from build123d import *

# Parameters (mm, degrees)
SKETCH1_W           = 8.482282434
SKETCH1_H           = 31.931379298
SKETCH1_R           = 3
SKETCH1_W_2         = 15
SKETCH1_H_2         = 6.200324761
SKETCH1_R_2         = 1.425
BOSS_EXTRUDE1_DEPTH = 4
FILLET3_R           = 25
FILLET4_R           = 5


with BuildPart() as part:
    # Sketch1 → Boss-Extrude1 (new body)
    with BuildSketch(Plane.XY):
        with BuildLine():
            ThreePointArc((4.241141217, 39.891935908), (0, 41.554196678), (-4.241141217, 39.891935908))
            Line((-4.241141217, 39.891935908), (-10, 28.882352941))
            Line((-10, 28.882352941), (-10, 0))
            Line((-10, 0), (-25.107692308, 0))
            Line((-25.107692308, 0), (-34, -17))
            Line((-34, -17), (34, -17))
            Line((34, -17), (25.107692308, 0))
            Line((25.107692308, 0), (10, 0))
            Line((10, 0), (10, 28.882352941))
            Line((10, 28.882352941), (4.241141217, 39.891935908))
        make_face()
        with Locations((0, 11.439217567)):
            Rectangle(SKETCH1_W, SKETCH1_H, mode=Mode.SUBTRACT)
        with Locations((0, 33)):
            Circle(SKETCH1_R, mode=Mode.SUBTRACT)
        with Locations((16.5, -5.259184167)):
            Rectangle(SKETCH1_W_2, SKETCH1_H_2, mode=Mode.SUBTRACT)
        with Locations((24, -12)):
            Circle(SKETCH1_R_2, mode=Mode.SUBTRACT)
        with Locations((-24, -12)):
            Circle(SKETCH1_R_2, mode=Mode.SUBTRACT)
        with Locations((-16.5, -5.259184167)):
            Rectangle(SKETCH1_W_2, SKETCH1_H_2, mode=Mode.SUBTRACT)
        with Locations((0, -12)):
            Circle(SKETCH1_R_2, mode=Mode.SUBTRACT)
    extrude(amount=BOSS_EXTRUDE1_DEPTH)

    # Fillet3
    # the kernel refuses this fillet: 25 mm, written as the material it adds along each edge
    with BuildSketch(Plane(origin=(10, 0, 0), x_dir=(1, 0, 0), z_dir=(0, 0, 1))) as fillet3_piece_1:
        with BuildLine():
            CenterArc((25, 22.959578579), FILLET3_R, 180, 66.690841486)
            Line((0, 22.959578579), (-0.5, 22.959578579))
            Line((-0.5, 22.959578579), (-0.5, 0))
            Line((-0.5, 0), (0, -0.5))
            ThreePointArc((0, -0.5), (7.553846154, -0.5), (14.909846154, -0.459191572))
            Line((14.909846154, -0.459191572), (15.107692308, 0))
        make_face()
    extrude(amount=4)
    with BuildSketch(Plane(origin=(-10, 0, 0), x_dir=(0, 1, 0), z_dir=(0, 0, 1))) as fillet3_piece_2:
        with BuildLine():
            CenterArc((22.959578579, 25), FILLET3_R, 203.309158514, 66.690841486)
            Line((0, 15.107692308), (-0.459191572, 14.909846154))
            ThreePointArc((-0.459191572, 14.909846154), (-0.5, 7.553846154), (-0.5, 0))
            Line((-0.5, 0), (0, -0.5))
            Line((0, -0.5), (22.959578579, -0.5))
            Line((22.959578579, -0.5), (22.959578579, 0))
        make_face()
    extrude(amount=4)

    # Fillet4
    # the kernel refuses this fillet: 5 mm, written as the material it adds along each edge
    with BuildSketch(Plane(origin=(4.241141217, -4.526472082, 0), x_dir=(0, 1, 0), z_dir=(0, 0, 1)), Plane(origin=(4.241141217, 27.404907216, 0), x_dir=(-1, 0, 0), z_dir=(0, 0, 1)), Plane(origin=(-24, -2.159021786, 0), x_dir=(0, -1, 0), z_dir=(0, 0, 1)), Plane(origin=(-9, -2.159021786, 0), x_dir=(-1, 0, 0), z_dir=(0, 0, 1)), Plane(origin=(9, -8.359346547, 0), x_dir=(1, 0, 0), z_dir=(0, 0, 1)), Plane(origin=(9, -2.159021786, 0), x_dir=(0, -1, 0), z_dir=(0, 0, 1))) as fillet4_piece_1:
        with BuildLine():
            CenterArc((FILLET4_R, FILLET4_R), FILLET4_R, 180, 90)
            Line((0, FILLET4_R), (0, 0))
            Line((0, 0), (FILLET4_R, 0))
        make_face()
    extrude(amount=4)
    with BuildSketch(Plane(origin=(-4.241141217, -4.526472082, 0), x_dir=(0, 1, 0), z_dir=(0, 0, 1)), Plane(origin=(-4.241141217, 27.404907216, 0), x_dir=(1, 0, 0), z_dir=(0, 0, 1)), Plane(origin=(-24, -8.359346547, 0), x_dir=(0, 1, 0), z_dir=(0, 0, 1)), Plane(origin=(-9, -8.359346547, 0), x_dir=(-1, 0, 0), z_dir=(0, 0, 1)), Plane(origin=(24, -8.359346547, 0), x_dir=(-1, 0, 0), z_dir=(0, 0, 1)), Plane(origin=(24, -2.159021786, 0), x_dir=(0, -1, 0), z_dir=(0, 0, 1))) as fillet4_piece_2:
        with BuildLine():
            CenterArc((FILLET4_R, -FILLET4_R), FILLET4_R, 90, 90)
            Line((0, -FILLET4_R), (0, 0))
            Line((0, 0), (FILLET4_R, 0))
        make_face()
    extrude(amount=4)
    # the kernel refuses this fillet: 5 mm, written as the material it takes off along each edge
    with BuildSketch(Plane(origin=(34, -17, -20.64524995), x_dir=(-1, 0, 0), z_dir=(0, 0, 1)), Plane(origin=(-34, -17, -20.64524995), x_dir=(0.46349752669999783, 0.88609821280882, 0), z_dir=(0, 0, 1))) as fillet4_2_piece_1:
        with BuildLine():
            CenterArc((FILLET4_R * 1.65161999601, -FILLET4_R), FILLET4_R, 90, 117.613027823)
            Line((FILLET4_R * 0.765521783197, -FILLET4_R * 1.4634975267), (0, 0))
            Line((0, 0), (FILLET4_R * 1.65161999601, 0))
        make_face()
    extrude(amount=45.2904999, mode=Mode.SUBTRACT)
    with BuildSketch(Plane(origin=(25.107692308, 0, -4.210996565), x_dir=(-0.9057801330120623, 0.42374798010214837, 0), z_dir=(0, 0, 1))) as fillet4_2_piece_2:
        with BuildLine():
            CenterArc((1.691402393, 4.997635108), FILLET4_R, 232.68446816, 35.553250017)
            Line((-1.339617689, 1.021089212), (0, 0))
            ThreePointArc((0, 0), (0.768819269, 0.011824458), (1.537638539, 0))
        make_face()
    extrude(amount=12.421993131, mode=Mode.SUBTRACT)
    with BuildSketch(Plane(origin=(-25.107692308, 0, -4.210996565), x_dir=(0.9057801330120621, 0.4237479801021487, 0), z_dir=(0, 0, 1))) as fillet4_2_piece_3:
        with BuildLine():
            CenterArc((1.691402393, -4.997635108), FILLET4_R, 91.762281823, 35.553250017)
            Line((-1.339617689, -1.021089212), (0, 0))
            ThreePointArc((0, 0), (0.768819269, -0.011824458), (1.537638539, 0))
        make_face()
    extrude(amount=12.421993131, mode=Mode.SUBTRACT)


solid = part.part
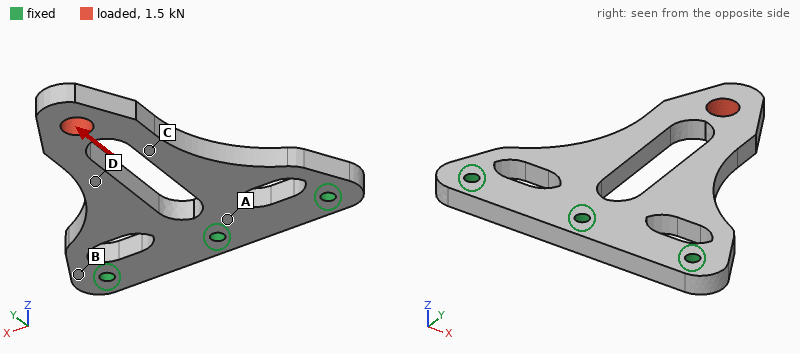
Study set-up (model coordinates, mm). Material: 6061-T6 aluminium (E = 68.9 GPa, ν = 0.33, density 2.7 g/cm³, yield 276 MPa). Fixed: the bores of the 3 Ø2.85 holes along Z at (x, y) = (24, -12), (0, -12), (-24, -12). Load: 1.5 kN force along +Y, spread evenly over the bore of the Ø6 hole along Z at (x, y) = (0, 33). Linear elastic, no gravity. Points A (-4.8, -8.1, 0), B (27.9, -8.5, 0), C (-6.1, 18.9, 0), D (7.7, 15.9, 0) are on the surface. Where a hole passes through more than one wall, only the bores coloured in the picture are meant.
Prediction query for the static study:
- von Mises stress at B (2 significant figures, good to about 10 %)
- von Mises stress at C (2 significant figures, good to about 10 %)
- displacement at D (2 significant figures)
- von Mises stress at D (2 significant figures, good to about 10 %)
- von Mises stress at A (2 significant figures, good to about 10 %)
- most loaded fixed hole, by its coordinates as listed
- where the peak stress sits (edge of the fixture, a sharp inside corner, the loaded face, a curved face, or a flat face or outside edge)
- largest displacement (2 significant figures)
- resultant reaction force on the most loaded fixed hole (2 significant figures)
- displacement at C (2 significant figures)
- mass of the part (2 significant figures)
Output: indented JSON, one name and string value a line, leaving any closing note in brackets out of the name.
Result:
{
  "von Mises stress at B": "10 MPa",
  "von Mises stress at C": "33 MPa",
  "displacement at D": "11 µm",
  "von Mises stress at D": "28 MPa",
  "von Mises stress at A": "18 MPa",
  "most loaded fixed hole, by its coordinates as listed": "(0, -12)",
  "where the peak stress sits": "a curved face",
  "largest displacement": "21 µm",
  "resultant reaction force on the most loaded fixed hole": "890 N",
  "displacement at C": "12 µm",
  "mass of the part": "16 g"
}
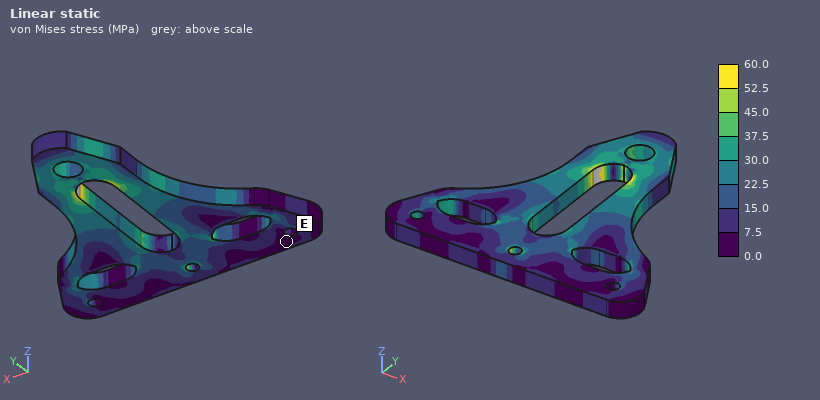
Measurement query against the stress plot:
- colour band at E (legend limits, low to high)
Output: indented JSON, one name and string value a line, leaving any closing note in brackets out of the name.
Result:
{
  "colour band at E": "0.0 to 7.5 MPa"
}
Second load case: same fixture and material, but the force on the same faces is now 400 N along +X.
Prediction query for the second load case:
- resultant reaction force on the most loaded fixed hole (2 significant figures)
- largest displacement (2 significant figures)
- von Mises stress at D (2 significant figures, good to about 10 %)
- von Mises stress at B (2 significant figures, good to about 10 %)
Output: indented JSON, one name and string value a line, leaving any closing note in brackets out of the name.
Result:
{
  "resultant reaction force on the most loaded fixed hole": "390 N",
  "largest displacement": "54 µm",
  "von Mises stress at D": "18 MPa",
  "von Mises stress at B": "12 MPa"
}
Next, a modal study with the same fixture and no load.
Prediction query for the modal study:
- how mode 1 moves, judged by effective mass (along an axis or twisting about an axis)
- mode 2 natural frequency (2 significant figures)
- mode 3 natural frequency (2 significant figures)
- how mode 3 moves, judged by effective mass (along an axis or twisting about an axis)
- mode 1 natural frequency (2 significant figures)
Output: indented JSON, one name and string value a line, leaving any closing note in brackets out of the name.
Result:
{
  "how mode 1 moves, judged by effective mass": "along Z",
  "mode 2 natural frequency": "6000 Hz",
  "mode 3 natural frequency": "7300 Hz",
  "how mode 3 moves, judged by effective mass": "along Z",
  "mode 1 natural frequency": "1500 Hz"
}
